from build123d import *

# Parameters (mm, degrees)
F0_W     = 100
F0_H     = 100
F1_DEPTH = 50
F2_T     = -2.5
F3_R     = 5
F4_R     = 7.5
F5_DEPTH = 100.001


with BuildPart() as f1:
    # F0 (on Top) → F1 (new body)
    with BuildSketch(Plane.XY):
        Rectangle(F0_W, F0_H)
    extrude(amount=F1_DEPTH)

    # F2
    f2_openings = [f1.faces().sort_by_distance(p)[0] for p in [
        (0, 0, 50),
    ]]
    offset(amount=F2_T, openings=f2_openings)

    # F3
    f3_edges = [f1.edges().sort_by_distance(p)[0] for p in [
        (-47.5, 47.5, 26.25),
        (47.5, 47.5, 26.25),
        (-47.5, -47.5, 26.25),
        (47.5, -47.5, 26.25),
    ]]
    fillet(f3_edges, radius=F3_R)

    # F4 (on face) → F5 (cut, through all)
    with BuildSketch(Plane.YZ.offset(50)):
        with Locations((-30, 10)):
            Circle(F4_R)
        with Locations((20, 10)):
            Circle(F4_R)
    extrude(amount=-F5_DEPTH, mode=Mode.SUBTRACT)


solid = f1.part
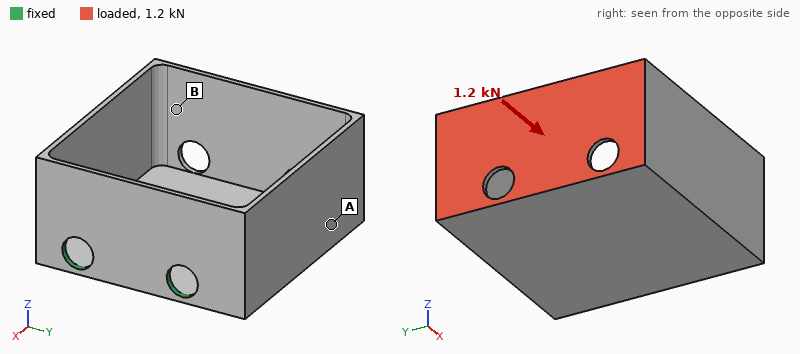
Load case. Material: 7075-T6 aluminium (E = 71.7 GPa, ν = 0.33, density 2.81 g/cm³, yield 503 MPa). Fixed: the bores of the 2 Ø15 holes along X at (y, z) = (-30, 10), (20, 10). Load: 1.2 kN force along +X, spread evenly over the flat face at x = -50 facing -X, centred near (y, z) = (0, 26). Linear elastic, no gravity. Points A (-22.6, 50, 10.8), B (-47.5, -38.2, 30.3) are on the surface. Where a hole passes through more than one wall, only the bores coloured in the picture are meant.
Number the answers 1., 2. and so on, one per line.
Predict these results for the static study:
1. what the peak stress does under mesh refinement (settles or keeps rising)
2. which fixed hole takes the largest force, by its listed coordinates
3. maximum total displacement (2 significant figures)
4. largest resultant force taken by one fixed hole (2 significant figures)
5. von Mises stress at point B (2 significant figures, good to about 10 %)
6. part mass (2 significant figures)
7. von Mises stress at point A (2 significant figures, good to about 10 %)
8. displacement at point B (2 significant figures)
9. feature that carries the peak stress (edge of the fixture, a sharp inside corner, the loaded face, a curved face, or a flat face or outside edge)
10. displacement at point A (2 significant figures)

1. keeps rising
2. (20, 10)
3. 1.5 mm
4. 780 N
5. 56 MPa
6. 200 g
7. 18 MPa
8. 0.84 mm
9. edge of the fixture
10. 0.82 mm
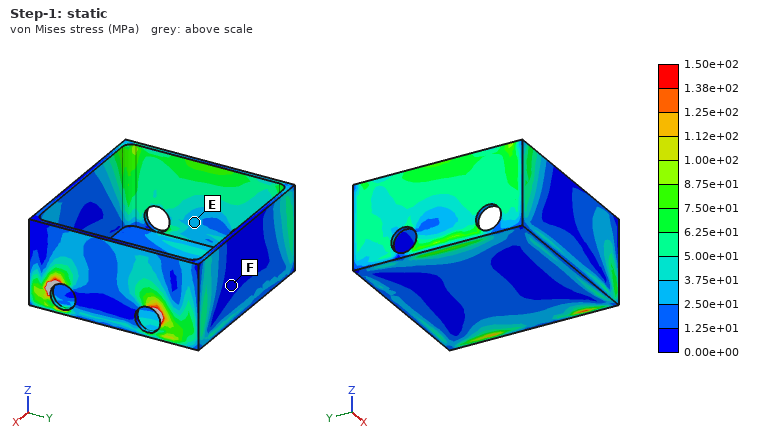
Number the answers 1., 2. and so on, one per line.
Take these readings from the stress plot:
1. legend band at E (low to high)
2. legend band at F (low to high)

1. 2.50e+01 to 3.75e+01 MPa
2. 0.00e+00 to 1.25e+01 MPa
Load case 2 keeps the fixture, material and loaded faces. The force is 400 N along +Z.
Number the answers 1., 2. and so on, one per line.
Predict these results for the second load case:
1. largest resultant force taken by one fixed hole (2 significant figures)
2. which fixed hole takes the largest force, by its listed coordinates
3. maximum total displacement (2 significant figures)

1. 270 N
2. (20, 10)
3. 1.7 mm
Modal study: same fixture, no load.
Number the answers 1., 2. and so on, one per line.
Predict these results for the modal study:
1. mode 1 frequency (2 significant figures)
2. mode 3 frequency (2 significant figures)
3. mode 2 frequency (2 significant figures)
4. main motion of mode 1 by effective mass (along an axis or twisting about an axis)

1. 300 Hz
2. 1400 Hz
3. 480 Hz
4. along Z
